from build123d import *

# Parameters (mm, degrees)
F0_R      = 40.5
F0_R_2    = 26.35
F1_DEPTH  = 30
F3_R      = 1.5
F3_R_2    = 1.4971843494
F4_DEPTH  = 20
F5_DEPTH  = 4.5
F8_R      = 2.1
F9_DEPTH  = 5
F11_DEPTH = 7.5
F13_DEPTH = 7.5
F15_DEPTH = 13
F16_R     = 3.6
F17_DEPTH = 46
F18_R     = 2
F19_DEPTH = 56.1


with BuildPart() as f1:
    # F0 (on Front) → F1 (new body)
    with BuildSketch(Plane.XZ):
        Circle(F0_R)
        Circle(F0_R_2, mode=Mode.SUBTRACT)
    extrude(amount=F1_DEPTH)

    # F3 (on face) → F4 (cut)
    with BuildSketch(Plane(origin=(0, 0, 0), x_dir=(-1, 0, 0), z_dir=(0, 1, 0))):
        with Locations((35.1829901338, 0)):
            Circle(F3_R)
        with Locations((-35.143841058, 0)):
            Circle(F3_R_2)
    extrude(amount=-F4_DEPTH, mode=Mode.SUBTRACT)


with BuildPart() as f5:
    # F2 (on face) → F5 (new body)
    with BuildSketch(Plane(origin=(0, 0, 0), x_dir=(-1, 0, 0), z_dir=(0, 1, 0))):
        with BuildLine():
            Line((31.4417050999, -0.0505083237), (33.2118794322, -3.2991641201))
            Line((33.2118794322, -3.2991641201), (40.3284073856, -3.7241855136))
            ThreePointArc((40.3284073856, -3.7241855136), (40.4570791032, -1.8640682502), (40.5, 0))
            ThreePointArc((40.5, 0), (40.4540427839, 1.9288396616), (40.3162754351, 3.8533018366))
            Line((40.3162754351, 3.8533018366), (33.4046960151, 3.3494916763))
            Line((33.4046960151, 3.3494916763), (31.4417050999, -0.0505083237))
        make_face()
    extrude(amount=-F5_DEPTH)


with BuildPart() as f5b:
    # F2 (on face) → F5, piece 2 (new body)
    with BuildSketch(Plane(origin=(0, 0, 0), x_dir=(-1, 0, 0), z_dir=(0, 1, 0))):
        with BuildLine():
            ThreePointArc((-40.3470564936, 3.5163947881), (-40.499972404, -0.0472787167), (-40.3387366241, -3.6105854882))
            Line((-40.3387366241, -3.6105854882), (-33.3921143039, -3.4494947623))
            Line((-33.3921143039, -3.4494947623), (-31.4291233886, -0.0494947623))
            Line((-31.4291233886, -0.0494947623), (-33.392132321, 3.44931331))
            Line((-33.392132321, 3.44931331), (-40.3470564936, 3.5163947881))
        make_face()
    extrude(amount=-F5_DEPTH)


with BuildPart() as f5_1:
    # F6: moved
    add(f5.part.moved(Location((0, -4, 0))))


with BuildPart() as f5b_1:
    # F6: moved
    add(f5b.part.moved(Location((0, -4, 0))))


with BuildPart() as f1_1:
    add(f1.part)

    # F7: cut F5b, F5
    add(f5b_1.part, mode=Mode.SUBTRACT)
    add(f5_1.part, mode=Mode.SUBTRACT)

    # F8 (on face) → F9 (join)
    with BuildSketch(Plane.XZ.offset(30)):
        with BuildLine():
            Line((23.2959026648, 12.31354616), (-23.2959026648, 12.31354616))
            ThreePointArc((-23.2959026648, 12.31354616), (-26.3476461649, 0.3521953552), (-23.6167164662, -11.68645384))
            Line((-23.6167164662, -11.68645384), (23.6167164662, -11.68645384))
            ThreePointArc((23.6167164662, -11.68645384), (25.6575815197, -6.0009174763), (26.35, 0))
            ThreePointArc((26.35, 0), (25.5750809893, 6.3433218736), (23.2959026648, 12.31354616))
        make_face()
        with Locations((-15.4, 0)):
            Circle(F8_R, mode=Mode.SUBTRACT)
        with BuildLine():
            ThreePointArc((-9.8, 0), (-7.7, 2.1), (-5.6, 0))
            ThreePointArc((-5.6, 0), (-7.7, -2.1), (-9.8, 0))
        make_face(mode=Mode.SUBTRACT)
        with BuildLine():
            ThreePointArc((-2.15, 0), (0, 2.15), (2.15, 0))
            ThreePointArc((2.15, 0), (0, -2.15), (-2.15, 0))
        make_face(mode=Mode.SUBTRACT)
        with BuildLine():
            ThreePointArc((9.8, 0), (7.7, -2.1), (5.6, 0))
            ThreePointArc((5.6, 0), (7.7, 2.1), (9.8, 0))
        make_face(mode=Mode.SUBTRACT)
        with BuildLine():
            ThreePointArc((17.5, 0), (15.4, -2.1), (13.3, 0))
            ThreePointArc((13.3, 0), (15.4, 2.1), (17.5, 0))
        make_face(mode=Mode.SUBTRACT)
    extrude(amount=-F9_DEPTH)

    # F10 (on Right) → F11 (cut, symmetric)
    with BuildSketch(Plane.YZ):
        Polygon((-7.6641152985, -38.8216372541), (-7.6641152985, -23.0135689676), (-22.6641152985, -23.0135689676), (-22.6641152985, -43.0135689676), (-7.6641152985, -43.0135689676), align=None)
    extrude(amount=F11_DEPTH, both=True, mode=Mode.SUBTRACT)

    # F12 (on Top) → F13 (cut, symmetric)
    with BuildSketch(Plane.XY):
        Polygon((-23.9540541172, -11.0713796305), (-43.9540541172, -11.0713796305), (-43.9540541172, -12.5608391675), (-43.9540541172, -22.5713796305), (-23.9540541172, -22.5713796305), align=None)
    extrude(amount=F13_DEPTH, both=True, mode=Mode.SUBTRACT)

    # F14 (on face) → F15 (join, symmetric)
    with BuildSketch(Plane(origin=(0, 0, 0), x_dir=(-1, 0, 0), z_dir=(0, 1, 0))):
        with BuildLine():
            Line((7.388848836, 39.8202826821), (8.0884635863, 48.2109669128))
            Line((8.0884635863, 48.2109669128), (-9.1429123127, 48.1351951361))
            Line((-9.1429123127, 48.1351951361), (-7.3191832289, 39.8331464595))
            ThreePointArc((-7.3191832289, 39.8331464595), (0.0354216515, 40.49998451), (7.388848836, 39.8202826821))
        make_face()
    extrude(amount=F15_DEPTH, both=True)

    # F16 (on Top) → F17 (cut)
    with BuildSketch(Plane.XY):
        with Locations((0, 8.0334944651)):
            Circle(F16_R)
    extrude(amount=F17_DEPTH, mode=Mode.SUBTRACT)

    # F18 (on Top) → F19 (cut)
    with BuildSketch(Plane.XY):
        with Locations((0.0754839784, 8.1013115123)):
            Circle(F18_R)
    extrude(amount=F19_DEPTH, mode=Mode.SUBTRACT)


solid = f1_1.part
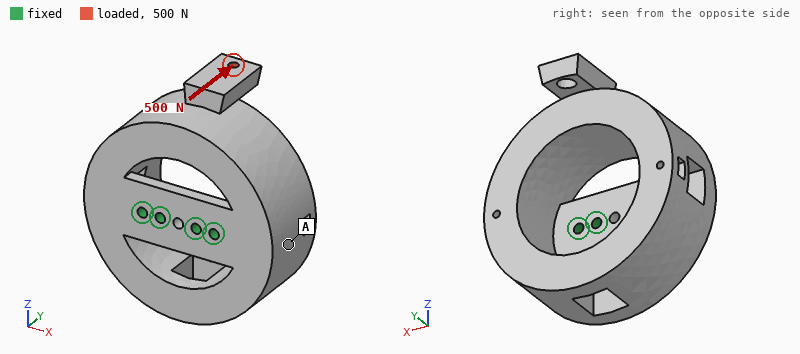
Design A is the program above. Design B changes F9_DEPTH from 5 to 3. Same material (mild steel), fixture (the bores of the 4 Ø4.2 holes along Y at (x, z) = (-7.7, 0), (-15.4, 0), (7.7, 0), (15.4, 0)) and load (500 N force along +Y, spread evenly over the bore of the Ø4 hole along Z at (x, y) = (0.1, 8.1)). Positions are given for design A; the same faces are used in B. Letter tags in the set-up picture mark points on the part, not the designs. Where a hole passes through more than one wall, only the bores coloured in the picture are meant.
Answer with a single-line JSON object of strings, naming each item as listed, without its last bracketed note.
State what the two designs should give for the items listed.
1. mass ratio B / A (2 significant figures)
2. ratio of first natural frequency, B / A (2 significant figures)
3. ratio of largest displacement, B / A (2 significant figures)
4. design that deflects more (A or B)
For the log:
{"mass ratio B / A": "0.97", "ratio of first natural frequency, B / A": "0.54", "ratio of largest displacement, B / A": "3.3", "design that deflects more": "B"}
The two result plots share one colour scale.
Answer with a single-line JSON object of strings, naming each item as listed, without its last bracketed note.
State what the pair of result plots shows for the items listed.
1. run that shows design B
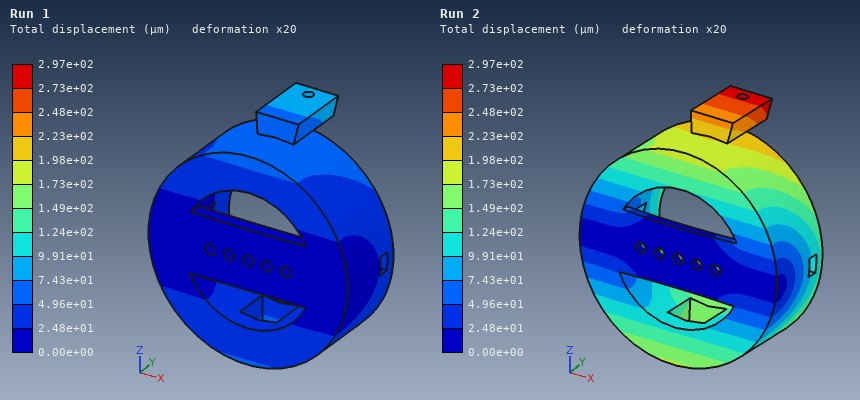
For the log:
{"run that shows design B": "Run 2"}
